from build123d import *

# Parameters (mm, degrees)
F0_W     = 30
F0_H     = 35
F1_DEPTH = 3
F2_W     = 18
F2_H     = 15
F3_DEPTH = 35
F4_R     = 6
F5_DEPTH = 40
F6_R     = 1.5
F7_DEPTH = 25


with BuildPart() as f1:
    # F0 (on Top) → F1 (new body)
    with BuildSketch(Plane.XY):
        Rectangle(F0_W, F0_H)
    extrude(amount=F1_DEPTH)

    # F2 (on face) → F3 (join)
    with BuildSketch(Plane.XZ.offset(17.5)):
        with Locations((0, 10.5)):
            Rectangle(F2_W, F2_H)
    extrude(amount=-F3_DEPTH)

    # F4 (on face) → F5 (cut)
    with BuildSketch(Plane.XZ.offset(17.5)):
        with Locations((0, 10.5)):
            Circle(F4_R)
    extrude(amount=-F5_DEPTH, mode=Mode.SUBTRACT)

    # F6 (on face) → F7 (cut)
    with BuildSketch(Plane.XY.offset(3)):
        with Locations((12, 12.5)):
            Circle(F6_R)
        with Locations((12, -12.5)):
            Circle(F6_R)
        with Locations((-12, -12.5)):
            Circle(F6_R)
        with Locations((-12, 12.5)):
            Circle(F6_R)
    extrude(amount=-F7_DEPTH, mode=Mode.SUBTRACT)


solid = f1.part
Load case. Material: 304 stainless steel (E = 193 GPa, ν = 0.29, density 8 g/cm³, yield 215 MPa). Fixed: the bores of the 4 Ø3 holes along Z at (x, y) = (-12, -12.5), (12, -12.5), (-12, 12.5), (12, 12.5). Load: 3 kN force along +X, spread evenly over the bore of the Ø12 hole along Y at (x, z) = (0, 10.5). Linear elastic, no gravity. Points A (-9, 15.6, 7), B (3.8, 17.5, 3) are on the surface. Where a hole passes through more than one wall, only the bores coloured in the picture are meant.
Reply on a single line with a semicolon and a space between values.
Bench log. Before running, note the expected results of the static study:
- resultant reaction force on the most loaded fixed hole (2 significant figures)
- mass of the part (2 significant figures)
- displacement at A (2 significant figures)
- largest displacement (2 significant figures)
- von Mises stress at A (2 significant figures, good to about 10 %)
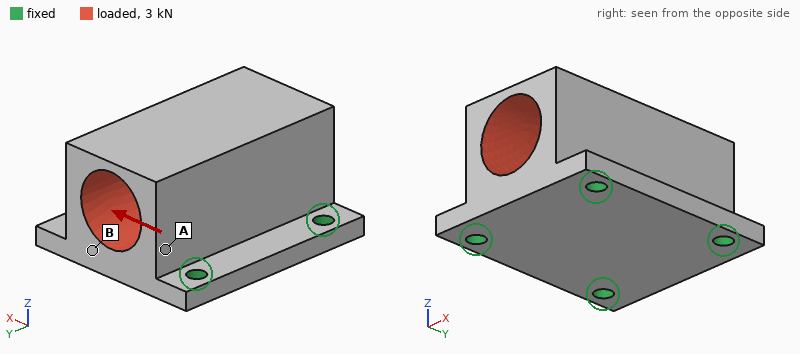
1.0 kN; 68 g; 3.3 µm; 11 µm; 41 MPa
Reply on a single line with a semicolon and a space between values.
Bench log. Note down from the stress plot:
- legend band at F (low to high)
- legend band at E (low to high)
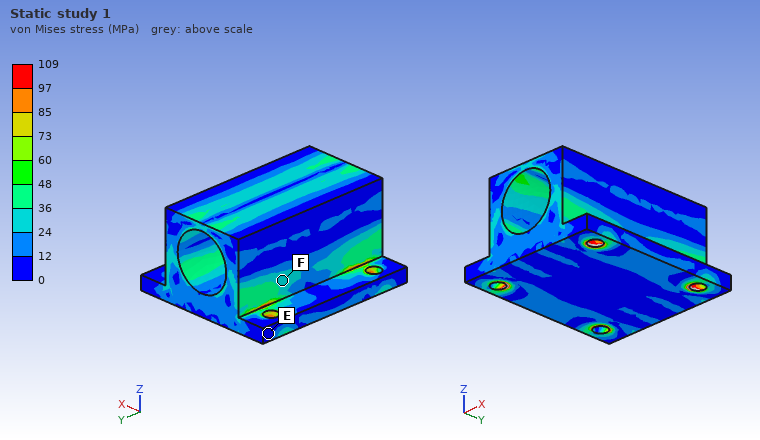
24 to 36 MPa; 0 to 12 MPa
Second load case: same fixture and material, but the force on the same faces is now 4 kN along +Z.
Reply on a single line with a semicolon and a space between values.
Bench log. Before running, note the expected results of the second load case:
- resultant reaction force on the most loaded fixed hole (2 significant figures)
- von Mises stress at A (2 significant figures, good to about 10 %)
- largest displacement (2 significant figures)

1.1 kN; 35 MPa; 5.5 µm
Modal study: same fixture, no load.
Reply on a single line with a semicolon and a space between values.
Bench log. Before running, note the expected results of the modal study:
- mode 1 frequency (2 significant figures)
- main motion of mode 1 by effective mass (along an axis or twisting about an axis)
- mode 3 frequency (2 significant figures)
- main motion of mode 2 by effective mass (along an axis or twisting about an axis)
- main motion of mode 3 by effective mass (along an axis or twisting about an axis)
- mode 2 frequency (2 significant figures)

14 kHz; along X; 19 kHz; along Y; along Z; 17 kHz
